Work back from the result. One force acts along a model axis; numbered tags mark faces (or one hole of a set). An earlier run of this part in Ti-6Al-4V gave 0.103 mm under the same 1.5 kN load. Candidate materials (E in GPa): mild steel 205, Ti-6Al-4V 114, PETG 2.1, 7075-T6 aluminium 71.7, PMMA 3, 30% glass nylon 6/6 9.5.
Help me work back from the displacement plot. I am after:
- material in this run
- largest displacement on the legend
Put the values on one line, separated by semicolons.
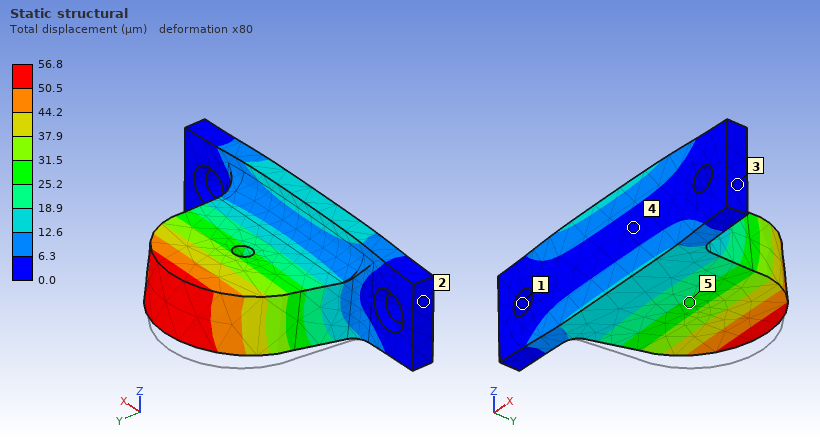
mild steel; 56.8 µm
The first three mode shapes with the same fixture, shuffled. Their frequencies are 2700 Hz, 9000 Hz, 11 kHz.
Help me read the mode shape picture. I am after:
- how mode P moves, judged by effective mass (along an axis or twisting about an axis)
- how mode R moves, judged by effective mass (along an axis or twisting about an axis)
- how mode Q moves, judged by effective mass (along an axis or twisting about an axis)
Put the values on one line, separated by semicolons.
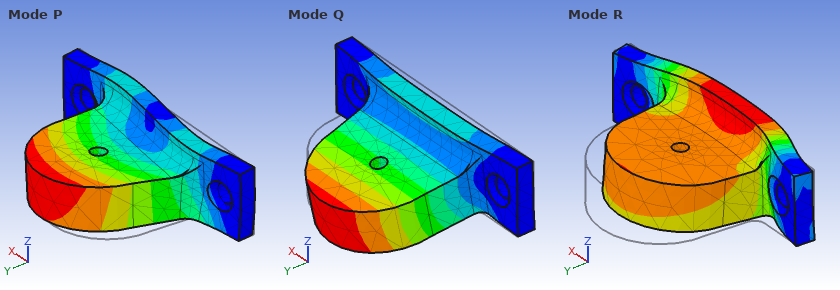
along X; along Y; along Z
